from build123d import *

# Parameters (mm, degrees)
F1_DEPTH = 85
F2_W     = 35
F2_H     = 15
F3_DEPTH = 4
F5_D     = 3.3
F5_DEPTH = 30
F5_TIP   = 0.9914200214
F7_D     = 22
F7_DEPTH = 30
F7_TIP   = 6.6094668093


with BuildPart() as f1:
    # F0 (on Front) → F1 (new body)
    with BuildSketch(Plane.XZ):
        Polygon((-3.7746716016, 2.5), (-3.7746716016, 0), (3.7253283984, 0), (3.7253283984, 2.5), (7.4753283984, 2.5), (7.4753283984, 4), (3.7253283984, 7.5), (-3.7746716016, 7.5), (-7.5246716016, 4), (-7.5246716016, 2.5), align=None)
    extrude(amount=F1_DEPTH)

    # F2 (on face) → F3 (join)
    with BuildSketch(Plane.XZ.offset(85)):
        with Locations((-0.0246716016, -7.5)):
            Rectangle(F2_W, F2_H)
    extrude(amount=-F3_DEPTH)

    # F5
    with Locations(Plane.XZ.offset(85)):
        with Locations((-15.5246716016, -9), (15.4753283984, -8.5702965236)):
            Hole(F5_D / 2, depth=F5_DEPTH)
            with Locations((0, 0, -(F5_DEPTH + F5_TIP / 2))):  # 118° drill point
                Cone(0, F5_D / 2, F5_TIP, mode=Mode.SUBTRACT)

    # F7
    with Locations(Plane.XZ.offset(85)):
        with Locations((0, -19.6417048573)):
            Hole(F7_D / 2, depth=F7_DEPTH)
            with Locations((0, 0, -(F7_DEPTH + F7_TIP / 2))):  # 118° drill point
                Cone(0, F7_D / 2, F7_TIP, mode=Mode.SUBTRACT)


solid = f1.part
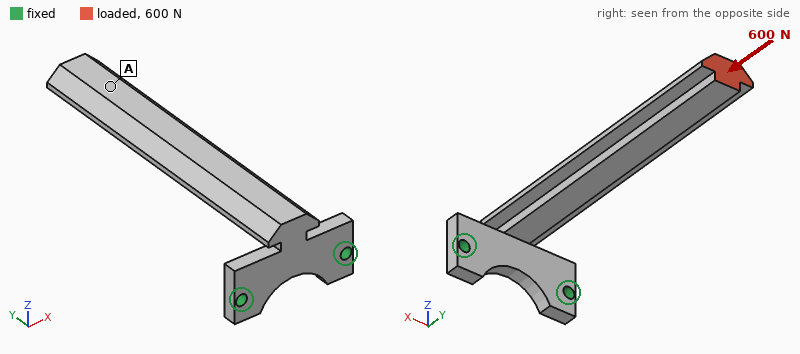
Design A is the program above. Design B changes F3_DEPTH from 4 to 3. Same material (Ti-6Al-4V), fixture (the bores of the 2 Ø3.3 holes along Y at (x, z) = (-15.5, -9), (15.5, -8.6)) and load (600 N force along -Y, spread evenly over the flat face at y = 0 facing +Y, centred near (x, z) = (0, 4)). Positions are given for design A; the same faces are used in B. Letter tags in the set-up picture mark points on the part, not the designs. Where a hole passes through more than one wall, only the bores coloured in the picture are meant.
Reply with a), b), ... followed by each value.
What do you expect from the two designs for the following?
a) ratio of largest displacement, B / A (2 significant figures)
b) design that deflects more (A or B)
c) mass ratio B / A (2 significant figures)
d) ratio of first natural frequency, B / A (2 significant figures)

a) 2.1
b) B
c) 0.95
d) 0.73
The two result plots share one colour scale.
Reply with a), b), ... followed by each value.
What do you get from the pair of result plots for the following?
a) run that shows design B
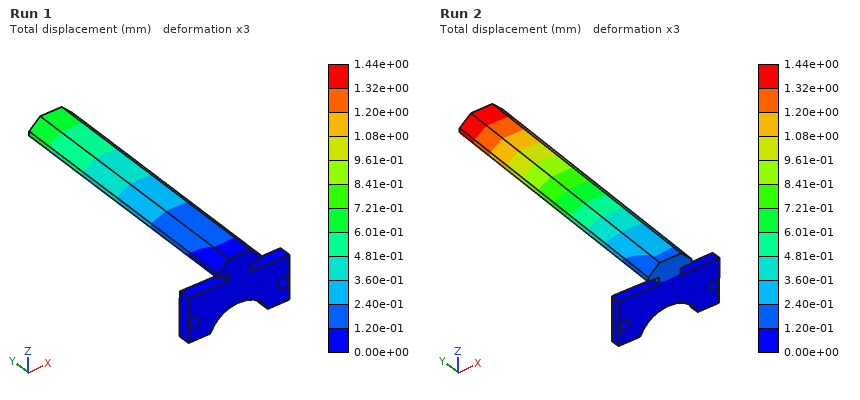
a) Run 2
